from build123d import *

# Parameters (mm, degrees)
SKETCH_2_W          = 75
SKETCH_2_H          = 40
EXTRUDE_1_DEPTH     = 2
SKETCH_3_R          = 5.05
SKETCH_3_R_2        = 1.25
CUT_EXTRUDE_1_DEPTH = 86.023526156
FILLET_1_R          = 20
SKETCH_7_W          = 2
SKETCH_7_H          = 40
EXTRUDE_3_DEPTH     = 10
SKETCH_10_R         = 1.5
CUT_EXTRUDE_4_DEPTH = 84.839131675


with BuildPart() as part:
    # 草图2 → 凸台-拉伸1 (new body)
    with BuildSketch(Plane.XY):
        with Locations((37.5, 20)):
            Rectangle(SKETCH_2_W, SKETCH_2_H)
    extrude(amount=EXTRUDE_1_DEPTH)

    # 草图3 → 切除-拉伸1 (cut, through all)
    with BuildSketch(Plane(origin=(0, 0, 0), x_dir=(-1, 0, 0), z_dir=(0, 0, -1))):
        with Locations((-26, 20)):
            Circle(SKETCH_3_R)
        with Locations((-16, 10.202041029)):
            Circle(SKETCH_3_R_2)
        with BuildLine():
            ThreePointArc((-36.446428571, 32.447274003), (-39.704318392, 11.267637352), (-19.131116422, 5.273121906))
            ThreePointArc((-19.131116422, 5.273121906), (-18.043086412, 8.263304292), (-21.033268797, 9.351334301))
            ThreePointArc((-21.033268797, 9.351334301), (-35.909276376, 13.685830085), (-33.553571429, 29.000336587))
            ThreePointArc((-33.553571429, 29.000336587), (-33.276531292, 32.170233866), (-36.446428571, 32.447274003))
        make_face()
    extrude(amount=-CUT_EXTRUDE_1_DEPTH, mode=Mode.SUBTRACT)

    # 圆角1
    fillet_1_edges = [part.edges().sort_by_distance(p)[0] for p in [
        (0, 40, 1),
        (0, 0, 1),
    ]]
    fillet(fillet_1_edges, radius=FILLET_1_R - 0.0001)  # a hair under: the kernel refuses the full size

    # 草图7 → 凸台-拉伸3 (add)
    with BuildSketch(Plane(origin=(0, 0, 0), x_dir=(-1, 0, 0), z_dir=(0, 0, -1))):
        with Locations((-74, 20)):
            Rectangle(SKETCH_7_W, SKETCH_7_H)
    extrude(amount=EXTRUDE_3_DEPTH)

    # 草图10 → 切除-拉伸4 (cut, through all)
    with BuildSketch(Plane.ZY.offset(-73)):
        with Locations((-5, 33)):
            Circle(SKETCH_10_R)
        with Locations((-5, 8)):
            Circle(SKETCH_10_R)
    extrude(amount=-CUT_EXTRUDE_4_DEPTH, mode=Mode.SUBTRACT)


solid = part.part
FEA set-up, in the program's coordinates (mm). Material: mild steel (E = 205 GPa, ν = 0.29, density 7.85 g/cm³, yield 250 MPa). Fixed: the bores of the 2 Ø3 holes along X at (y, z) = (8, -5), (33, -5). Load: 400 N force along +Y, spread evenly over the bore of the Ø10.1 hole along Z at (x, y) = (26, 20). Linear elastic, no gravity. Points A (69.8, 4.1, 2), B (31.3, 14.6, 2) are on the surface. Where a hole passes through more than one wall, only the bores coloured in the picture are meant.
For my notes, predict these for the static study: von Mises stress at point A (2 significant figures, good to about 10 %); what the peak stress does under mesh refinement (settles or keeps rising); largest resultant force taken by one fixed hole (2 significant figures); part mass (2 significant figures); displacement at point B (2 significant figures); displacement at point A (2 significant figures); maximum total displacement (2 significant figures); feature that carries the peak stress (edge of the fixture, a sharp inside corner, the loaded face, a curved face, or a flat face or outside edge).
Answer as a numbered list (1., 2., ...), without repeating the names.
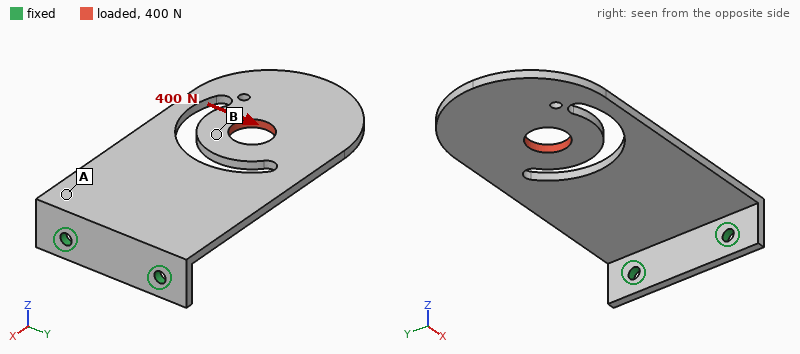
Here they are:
1. 57 MPa
2. keeps rising
3. 750 N
4. 46 g
5. 0.079 mm
6. 0.030 mm
7. 0.13 mm
8. edge of the fixture
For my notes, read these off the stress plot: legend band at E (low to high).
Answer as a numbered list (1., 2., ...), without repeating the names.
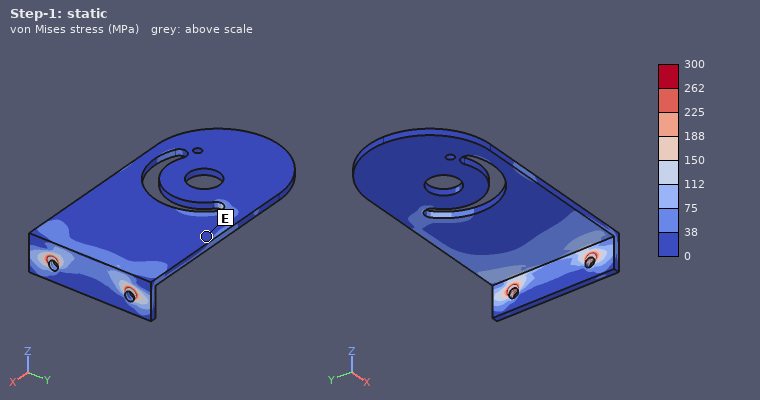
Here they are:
1. 0 to 38 MPa
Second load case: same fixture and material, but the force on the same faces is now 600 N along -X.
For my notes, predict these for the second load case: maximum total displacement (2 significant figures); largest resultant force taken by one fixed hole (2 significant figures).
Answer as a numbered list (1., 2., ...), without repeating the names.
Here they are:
1. 0.16 mm
2. 310 N
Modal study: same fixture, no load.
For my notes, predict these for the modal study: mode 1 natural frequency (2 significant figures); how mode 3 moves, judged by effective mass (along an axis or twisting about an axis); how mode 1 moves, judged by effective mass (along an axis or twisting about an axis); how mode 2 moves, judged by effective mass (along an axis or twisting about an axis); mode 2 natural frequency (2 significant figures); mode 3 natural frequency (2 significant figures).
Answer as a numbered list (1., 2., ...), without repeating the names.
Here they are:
1. 290 Hz
2. along Z
3. along Z
4. twisting about X
5. 1200 Hz
6. 1400 Hz
